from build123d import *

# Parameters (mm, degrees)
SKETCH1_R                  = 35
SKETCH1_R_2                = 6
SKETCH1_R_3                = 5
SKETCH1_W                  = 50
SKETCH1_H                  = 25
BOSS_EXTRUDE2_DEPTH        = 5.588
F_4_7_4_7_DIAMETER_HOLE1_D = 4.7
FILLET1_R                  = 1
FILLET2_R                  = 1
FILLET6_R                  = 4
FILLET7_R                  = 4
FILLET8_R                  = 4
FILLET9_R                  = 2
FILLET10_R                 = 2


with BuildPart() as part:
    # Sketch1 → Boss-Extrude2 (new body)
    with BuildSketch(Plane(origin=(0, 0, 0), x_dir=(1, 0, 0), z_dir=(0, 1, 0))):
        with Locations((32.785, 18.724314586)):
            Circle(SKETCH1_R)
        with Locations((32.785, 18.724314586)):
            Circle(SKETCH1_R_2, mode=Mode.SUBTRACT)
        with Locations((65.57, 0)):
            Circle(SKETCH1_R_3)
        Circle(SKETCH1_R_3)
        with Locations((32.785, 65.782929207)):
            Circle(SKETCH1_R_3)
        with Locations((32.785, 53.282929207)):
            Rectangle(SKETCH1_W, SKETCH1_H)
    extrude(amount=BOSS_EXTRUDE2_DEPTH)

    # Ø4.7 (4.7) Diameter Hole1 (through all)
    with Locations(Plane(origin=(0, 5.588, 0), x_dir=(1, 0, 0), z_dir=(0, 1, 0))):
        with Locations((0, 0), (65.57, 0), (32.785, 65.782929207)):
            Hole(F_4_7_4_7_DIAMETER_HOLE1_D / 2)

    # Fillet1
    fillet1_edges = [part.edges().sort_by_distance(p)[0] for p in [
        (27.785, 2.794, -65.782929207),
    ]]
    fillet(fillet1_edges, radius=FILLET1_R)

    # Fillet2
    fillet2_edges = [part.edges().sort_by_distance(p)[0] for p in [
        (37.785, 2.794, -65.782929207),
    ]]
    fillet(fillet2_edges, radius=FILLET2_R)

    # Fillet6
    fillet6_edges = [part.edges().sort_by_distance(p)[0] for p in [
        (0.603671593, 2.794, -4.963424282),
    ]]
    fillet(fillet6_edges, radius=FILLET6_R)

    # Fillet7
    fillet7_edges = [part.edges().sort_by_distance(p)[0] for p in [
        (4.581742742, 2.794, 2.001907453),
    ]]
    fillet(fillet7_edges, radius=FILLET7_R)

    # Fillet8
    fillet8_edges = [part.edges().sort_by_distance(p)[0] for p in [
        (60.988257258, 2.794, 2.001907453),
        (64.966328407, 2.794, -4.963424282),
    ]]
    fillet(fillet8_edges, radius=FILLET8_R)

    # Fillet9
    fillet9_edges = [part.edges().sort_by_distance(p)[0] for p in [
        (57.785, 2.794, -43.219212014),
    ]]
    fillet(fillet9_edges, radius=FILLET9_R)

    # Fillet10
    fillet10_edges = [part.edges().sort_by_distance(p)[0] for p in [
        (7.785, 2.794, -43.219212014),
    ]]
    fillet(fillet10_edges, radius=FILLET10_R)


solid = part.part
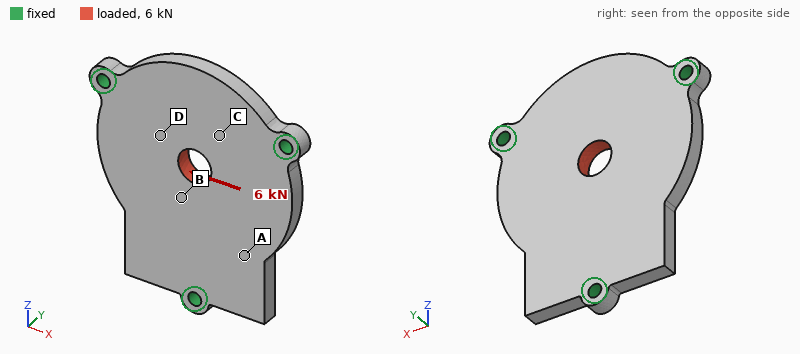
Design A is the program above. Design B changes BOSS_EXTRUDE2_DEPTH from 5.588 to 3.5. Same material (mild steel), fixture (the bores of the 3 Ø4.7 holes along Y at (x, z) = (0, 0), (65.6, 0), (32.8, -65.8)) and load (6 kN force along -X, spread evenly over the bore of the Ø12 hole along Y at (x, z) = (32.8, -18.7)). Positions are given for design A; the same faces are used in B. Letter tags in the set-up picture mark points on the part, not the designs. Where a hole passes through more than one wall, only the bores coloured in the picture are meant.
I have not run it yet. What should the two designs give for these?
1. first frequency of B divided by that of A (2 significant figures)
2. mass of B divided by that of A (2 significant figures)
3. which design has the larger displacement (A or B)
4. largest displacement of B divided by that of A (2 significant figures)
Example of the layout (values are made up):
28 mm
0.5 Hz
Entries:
0.66
0.63
B
1.6
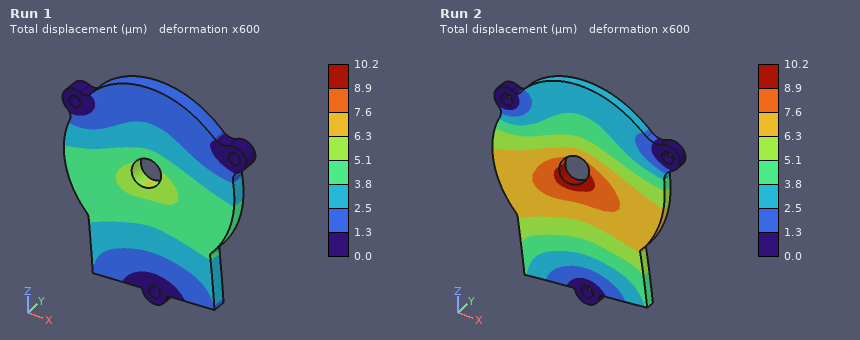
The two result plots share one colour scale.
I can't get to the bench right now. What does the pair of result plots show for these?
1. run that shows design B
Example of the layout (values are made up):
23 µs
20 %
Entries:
Run 2
